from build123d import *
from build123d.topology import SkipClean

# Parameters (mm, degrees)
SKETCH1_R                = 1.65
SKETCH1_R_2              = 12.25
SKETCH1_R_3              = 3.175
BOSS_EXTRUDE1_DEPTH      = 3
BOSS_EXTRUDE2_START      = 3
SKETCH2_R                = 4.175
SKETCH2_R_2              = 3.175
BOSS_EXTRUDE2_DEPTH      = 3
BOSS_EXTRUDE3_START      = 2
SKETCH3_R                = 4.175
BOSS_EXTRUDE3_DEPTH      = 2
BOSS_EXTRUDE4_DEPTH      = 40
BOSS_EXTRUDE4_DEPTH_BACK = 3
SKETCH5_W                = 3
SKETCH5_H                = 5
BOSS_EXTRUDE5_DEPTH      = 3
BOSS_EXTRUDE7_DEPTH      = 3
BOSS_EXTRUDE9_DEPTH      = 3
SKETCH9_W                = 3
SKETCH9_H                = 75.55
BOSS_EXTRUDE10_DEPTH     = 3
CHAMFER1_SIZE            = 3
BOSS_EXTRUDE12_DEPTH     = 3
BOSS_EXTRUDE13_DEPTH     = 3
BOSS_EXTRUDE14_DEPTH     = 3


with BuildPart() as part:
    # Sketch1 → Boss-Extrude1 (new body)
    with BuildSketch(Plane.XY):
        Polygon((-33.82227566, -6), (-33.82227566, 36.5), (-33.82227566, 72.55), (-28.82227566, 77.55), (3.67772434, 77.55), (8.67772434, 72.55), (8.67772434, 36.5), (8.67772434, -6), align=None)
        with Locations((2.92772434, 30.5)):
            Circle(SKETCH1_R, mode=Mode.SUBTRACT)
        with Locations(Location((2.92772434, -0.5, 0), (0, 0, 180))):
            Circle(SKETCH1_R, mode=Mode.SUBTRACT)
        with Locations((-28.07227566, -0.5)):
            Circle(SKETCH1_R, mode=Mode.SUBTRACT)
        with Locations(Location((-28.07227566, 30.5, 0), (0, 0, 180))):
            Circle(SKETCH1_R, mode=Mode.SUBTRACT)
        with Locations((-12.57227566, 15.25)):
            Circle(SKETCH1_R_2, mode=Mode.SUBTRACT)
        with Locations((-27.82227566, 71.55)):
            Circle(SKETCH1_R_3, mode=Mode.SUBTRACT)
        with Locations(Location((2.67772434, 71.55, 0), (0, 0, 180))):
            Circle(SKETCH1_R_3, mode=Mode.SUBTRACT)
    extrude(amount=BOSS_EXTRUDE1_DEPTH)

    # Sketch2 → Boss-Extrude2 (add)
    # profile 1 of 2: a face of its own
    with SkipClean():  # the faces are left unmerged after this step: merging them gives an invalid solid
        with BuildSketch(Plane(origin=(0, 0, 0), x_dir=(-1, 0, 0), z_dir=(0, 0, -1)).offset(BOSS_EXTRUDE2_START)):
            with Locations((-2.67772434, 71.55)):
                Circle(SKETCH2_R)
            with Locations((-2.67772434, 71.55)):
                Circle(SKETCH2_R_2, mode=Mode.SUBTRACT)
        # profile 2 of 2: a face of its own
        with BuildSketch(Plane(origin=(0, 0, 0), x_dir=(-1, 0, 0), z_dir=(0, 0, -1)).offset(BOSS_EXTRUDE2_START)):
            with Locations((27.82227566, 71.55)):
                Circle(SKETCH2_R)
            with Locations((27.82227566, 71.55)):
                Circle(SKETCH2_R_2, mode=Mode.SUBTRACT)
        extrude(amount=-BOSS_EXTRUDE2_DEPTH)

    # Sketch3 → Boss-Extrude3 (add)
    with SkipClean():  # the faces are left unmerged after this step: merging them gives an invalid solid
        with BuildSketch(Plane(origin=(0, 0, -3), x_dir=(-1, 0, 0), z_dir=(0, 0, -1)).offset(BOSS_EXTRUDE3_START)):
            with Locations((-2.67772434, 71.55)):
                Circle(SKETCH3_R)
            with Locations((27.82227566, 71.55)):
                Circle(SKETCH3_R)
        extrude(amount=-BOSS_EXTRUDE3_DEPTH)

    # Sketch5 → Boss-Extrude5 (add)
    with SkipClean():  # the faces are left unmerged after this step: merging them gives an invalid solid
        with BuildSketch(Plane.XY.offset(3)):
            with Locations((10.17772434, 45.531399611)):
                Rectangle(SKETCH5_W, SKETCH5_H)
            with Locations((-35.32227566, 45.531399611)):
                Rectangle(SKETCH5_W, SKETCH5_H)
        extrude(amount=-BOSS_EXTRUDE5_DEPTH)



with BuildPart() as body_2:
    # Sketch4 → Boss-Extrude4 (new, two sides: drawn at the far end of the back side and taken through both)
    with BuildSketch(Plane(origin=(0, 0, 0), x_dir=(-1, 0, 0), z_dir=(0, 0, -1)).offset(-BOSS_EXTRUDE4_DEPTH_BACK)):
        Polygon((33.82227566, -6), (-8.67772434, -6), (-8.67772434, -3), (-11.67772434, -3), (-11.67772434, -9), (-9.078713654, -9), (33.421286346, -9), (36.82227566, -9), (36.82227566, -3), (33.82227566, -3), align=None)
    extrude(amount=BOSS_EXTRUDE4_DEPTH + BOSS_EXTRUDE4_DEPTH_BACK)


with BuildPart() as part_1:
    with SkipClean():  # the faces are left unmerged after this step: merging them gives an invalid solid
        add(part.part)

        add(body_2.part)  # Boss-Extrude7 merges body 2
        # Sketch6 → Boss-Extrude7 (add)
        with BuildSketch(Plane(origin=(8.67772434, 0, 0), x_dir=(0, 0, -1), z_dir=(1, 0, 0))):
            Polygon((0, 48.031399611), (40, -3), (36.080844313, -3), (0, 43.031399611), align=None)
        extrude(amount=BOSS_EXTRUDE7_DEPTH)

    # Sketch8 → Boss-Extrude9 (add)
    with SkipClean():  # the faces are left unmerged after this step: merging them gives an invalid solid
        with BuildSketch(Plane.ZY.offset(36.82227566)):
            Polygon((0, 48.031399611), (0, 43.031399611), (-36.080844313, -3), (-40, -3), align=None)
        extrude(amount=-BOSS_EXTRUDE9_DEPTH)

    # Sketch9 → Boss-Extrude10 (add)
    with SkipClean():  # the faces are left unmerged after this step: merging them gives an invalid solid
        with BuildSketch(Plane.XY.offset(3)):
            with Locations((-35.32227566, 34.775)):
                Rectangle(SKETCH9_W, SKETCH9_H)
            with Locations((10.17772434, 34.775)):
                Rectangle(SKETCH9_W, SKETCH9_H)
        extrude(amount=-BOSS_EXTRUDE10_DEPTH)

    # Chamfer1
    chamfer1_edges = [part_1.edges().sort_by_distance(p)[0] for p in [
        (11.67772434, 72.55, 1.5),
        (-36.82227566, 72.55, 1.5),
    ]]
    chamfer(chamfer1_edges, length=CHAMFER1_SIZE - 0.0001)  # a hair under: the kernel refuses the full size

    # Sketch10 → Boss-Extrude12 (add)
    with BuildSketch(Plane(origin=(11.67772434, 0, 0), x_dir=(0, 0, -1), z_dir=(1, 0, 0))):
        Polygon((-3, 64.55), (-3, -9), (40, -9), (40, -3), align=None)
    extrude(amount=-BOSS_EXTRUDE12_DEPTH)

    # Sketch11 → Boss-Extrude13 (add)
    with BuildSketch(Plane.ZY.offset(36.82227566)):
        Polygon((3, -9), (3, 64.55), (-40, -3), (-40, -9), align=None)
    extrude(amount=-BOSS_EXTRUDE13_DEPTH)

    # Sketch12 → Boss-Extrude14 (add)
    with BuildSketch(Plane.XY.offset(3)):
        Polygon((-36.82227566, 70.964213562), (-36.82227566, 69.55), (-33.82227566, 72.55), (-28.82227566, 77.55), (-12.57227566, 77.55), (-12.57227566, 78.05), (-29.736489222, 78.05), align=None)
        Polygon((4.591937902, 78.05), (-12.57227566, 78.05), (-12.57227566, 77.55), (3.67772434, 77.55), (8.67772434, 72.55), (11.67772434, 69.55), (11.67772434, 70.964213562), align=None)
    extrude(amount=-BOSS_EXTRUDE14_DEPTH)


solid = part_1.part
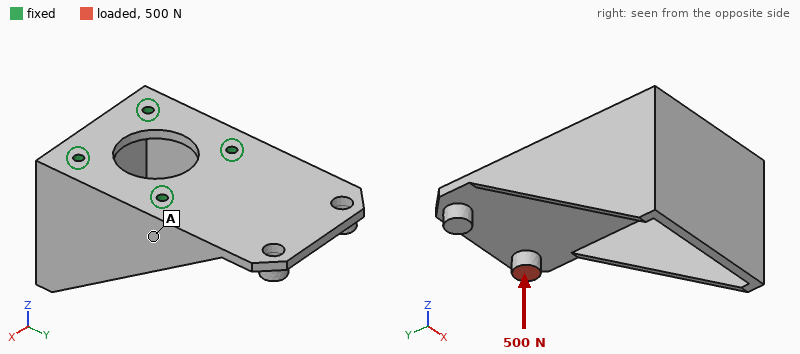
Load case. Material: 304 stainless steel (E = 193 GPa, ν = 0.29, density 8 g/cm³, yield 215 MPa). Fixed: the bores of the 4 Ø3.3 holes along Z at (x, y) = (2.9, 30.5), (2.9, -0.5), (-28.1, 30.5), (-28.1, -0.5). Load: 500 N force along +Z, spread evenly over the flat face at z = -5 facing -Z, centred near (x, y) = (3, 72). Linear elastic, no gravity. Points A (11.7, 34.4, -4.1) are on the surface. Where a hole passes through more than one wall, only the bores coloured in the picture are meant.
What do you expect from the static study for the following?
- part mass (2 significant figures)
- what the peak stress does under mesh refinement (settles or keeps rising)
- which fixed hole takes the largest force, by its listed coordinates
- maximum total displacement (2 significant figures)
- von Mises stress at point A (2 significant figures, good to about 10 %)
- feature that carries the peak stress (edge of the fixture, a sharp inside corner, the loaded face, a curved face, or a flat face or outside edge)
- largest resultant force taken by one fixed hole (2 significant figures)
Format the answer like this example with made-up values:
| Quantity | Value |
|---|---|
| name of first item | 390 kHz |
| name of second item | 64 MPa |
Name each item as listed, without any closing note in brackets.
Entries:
| Quantity | Value |
|---|---|
| part mass | 200 g |
| what the peak stress does under mesh refinement | keeps rising |
| which fixed hole takes the largest force, by its listed coordinates | (2.9, 30.5) |
| maximum total displacement | 0.21 mm |
| von Mises stress at point A | 27 MPa |
| feature that carries the peak stress | edge of the fixture |
| largest resultant force taken by one fixed hole | 960 N |
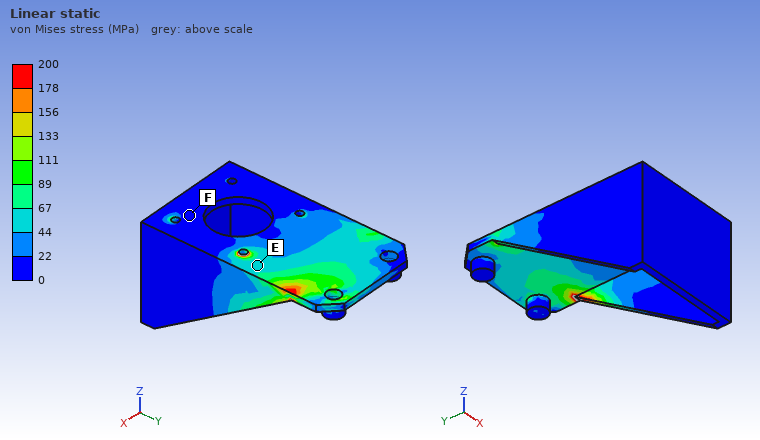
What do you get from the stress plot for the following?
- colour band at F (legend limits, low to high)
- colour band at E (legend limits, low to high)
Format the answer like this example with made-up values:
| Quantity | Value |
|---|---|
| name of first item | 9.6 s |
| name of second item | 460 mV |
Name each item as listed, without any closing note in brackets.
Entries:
| Quantity | Value |
|---|---|
| colour band at F | 0 to 22 MPa |
| colour band at E | 44 to 67 MPa |
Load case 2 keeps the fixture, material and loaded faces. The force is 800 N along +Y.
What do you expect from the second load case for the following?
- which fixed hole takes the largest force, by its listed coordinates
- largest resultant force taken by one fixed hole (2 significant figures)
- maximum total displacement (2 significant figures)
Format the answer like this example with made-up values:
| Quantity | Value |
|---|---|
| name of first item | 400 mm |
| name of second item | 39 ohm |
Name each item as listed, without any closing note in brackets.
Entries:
| Quantity | Value |
|---|---|
| which fixed hole takes the largest force, by its listed coordinates | (2.9, 30.5) |
| largest resultant force taken by one fixed hole | 560 N |
| maximum total displacement | 0.13 mm |
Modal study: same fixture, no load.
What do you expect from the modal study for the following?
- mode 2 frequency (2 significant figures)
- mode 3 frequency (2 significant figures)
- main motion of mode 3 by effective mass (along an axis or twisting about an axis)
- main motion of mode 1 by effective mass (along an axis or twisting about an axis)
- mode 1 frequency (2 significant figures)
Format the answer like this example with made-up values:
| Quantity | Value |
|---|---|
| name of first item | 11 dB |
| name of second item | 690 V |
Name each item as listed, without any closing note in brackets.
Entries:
| Quantity | Value |
|---|---|
| mode 2 frequency | 3700 Hz |
| mode 3 frequency | 4100 Hz |
| main motion of mode 3 by effective mass | along X |
| main motion of mode 1 by effective mass | along Z |
| mode 1 frequency | 2300 Hz |
